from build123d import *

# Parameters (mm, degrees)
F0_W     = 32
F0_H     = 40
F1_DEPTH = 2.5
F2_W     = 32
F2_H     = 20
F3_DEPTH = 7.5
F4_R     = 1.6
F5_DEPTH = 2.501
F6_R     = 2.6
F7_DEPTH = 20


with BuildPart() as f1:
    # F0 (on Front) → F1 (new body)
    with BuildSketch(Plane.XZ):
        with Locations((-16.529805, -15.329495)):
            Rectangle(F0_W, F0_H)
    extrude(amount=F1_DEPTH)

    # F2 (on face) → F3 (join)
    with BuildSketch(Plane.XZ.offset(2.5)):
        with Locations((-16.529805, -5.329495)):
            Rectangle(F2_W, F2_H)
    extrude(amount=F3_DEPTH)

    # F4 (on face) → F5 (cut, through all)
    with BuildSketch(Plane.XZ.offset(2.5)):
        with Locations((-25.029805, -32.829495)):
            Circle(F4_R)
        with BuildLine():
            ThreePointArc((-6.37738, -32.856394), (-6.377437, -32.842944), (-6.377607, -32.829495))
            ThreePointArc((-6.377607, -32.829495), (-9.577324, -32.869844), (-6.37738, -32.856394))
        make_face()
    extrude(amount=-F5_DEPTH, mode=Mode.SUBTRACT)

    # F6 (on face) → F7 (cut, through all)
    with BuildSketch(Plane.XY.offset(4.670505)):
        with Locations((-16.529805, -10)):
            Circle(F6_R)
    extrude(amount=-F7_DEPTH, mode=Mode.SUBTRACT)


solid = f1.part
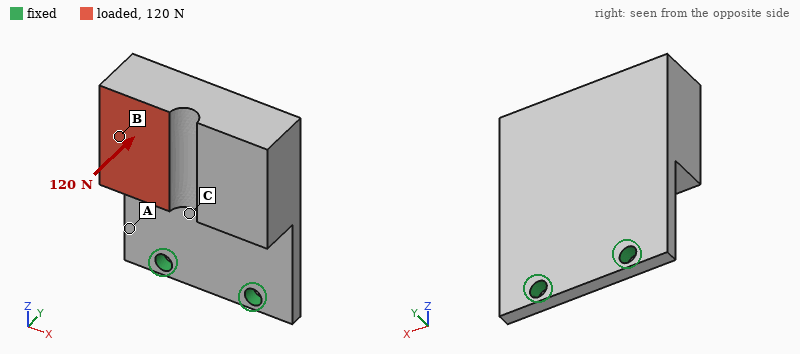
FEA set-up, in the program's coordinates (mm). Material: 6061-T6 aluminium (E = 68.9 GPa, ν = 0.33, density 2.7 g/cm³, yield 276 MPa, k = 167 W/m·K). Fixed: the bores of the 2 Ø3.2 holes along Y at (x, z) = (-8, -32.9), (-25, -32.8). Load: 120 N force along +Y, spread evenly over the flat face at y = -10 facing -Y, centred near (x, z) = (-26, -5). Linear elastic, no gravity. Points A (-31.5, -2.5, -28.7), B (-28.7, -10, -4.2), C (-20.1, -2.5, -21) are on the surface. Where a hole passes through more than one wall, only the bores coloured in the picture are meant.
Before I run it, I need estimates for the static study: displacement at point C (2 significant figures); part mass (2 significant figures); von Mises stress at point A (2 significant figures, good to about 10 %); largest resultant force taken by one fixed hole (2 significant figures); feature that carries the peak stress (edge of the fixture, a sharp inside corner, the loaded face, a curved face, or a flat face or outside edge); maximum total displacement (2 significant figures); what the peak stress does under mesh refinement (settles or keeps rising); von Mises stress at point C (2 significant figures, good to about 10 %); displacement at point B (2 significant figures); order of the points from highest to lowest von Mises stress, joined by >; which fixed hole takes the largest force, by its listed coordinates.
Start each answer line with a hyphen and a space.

- 0.076 mm
- 21 g
- 83 MPa
- 110 N
- edge of the fixture
- 0.46 mm
- keeps rising
- 51 MPa
- 0.33 mm
- A > C > B
- (-25, -32.8)
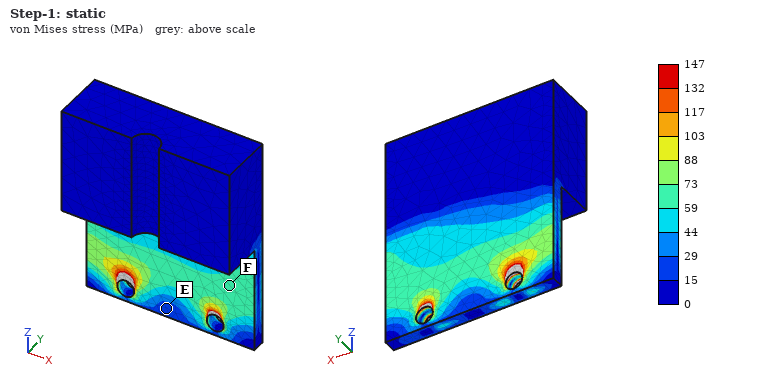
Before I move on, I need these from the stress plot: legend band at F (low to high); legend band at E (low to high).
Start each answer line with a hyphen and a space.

- 59 to 73 MPa
- 15 to 29 MPa
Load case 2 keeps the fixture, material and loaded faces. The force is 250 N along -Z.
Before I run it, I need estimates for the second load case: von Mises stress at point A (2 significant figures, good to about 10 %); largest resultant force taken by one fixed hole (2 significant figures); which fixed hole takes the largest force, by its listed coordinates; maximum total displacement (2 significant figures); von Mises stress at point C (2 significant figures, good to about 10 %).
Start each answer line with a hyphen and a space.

- 60 MPa
- 250 N
- (-25, -32.8)
- 0.41 mm
- 64 MPa
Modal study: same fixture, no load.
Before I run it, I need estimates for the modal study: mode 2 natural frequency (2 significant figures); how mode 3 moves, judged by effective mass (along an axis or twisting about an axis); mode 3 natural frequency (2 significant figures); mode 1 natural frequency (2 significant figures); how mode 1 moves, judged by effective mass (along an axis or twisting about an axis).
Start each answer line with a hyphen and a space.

- 2800 Hz
- along X
- 6000 Hz
- 760 Hz
- along Y
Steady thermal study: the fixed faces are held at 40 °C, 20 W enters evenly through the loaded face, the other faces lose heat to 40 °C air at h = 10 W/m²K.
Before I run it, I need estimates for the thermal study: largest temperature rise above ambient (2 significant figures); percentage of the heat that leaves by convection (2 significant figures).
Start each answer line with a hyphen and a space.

- 38 K
- 4.1 %
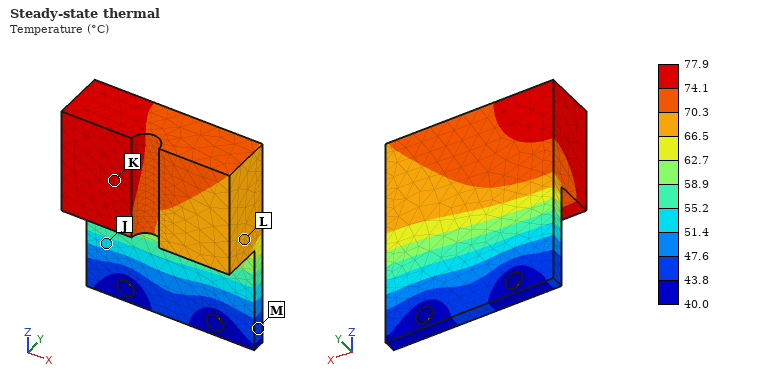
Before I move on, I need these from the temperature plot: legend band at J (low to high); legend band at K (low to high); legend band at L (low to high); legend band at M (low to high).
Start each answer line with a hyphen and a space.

- 51.4 to 55.2 °C
- 74.1 to 77.9 °C
- 66.5 to 70.3 °C
- 43.8 to 47.6 °C
